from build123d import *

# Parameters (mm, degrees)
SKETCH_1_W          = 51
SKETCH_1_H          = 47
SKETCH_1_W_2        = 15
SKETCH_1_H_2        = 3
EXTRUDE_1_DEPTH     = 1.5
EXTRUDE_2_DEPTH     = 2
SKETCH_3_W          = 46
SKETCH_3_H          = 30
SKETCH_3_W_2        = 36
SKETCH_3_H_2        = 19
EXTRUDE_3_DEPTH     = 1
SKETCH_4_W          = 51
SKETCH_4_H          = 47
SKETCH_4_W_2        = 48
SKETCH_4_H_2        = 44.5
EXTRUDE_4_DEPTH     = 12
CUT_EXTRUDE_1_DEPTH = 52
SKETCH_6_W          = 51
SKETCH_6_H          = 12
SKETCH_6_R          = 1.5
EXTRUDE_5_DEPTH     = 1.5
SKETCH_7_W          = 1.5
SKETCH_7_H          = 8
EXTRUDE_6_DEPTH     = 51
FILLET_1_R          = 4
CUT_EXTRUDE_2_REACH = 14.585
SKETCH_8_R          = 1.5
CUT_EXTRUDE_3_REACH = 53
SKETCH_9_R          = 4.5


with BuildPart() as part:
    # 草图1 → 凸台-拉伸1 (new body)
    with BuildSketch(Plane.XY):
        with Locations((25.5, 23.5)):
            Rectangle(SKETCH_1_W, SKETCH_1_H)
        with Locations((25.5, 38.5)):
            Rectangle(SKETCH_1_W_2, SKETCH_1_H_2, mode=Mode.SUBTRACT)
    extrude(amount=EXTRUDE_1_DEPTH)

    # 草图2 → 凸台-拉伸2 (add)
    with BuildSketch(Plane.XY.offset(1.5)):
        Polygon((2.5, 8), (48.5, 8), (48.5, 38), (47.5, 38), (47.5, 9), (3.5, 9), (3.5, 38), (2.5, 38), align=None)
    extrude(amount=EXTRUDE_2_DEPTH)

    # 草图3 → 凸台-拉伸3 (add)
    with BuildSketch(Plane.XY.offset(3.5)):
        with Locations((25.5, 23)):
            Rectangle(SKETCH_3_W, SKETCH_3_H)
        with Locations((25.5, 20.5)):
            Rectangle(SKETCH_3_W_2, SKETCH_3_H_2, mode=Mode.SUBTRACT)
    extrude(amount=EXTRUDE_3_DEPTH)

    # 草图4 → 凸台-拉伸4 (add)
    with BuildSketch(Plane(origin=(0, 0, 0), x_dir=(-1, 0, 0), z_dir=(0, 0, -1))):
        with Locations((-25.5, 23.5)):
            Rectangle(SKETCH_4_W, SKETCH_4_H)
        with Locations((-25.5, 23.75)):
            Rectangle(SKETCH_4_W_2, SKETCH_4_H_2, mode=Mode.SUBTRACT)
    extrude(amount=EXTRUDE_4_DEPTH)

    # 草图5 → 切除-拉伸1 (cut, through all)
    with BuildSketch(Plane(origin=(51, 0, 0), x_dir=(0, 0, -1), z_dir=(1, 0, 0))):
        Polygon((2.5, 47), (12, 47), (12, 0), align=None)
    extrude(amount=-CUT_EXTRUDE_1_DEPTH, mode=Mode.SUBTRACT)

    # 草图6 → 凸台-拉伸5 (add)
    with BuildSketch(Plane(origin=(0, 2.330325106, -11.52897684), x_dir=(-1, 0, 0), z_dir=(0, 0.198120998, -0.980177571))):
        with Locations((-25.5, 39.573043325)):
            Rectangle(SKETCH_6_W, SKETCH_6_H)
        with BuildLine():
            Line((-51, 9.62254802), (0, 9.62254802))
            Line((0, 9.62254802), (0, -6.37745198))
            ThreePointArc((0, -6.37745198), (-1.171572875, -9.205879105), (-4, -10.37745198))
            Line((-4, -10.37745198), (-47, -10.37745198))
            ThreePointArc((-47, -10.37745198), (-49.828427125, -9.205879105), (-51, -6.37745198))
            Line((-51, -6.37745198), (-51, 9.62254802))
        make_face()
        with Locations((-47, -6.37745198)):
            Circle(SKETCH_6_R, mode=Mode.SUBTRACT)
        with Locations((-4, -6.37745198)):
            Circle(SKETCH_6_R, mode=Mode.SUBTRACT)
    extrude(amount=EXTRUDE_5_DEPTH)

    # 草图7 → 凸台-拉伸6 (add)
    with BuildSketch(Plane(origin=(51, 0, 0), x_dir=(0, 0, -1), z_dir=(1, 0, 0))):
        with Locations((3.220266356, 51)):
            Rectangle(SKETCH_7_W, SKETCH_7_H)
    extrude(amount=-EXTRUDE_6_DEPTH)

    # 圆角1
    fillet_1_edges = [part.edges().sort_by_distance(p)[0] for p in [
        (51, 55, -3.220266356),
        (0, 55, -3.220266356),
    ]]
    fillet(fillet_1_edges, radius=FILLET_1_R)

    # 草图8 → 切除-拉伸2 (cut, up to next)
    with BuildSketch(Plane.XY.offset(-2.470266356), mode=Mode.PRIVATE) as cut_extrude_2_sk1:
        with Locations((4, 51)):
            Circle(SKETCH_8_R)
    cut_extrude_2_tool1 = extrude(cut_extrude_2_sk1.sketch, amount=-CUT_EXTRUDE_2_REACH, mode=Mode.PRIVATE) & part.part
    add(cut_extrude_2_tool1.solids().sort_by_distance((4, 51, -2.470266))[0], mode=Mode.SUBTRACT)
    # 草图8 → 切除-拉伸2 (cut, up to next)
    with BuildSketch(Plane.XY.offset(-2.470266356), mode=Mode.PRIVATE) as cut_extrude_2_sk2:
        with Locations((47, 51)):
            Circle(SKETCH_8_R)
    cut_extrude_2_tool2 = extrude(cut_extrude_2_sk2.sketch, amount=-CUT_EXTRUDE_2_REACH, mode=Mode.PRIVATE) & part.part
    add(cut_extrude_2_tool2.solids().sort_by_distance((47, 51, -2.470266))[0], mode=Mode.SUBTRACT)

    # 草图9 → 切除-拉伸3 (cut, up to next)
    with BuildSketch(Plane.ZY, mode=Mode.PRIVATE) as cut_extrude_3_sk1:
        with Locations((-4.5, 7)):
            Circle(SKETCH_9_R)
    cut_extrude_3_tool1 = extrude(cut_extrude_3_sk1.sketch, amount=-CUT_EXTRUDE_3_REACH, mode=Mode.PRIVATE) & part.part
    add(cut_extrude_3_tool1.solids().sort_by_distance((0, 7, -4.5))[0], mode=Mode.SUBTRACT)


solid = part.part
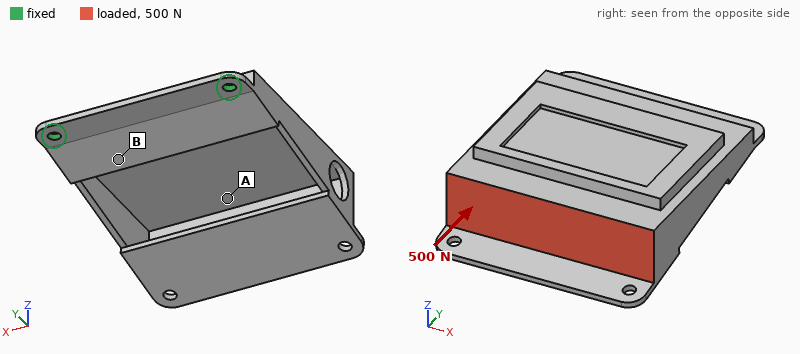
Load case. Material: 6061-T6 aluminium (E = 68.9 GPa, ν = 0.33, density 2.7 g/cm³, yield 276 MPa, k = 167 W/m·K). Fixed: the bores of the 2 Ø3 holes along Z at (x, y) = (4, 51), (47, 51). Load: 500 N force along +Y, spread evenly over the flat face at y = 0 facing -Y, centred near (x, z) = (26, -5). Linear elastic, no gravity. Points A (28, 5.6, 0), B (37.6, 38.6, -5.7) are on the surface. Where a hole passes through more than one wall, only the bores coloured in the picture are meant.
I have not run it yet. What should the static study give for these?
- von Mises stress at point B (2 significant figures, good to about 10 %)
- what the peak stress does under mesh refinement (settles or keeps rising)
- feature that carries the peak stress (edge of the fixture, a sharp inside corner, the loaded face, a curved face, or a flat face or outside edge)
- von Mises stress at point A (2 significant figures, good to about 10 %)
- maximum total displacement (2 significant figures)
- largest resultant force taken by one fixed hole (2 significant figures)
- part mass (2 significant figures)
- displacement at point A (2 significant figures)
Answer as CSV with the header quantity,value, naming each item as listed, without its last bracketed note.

quantity,value
von Mises stress at point B,7.8 MPa
what the peak stress does under mesh refinement,keeps rising
feature that carries the peak stress,edge of the fixture
von Mises stress at point A,15 MPa
maximum total displacement,0.65 mm
largest resultant force taken by one fixed hole,260 N
part mass,25 g
displacement at point A,0.47 mm
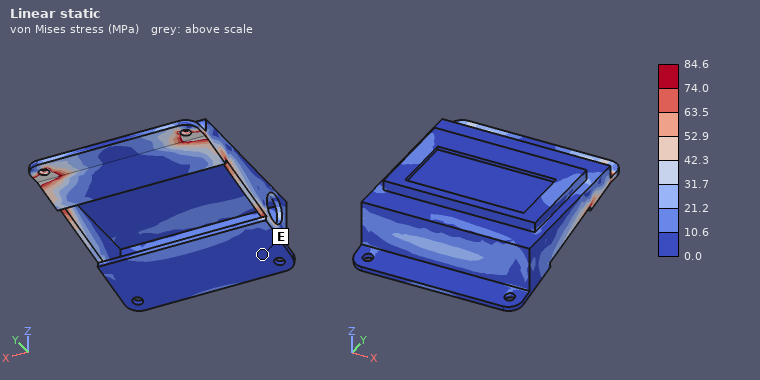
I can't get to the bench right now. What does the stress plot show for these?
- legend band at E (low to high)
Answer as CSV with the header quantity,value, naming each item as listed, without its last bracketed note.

quantity,value
legend band at E,0.0 to 10.6 MPa
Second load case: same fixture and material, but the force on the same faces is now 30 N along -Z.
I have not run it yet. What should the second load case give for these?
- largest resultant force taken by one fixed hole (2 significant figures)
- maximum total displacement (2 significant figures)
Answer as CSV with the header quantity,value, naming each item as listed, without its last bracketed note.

quantity,value
largest resultant force taken by one fixed hole,41 N
maximum total displacement,0.76 mm
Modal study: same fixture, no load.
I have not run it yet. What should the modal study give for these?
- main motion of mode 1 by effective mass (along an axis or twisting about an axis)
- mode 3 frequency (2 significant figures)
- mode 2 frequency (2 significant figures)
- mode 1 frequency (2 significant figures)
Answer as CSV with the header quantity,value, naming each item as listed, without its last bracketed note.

quantity,value
main motion of mode 1 by effective mass,along Z
mode 3 frequency,2600 Hz
mode 2 frequency,1000 Hz
mode 1 frequency,320 Hz
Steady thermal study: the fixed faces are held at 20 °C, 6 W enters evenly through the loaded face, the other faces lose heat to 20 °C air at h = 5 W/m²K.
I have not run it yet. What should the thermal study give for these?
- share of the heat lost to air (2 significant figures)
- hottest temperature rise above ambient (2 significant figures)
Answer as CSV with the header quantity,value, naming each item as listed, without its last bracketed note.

quantity,value
share of the heat lost to air,14 %
hottest temperature rise above ambient,21 K
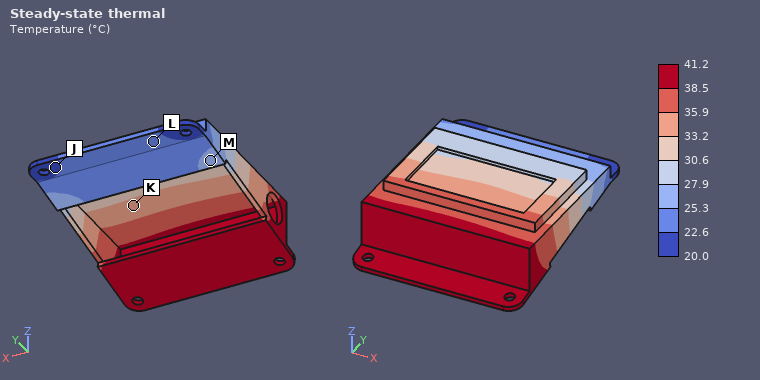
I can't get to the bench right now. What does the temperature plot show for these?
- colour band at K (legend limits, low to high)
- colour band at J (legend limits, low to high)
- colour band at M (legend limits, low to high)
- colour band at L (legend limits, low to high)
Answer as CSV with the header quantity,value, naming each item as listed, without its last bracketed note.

quantity,value
colour band at K,33.2 to 35.9 °C
colour band at J,20.0 to 22.6 °C
colour band at M,25.3 to 27.9 °C
colour band at L,22.6 to 25.3 °C
